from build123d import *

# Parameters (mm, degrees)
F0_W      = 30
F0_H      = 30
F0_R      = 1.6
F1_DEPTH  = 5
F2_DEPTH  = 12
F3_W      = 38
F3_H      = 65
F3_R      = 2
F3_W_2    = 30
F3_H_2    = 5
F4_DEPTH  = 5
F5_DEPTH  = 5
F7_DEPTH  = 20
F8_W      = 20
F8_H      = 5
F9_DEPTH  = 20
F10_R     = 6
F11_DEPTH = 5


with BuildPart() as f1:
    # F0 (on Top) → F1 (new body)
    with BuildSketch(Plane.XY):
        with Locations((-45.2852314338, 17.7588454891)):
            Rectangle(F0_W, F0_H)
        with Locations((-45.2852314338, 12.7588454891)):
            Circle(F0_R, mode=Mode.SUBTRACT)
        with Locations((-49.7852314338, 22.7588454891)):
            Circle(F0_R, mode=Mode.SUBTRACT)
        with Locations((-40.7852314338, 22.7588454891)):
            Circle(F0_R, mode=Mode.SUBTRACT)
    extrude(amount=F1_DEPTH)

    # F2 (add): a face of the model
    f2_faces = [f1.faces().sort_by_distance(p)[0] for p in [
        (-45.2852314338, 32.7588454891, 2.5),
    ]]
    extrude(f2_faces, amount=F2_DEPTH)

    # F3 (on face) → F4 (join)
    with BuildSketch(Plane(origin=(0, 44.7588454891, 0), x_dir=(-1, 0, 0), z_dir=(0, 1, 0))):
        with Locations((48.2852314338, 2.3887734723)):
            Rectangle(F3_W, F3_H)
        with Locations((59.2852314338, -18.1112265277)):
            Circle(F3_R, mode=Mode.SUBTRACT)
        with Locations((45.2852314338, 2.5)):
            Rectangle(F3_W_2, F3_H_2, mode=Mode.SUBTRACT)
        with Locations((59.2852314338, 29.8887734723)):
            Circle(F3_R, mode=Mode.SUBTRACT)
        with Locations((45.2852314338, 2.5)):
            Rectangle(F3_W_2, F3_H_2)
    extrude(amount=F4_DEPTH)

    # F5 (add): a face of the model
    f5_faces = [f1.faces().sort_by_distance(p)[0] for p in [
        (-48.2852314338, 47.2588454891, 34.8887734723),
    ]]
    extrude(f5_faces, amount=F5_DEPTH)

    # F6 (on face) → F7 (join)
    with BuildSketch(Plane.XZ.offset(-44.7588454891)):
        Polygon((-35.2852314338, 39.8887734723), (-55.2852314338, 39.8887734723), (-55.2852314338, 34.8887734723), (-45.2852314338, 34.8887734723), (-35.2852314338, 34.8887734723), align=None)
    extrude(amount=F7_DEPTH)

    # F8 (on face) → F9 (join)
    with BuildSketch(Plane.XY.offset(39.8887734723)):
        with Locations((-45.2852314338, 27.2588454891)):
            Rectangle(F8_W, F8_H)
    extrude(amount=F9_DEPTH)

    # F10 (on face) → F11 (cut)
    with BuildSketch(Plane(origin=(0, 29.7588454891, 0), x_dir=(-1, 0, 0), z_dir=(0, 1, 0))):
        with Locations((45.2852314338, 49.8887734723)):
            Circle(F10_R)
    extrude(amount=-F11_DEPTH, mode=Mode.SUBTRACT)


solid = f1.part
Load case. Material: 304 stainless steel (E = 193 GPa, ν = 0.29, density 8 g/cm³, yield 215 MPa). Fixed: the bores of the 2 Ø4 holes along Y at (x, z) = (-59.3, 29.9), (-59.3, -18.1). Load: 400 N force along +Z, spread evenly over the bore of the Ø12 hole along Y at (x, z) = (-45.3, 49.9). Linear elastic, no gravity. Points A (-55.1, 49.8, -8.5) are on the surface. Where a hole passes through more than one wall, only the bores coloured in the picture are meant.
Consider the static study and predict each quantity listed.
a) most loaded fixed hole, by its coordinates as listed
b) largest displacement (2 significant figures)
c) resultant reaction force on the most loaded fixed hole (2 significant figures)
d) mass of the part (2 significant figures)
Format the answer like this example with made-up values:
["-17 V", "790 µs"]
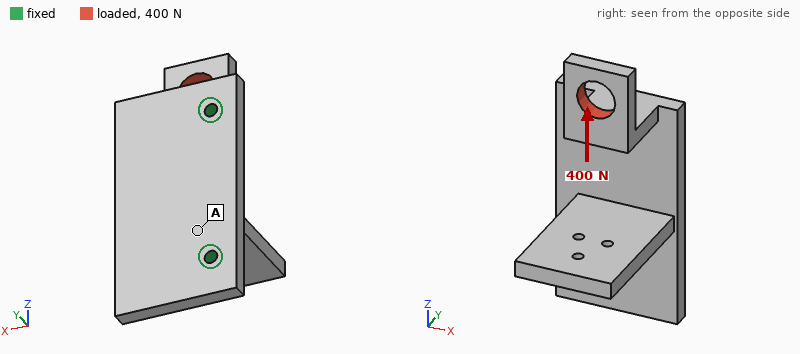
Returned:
["(-59.3, 29.9)", "0.11 mm", "290 N", "180 g"]
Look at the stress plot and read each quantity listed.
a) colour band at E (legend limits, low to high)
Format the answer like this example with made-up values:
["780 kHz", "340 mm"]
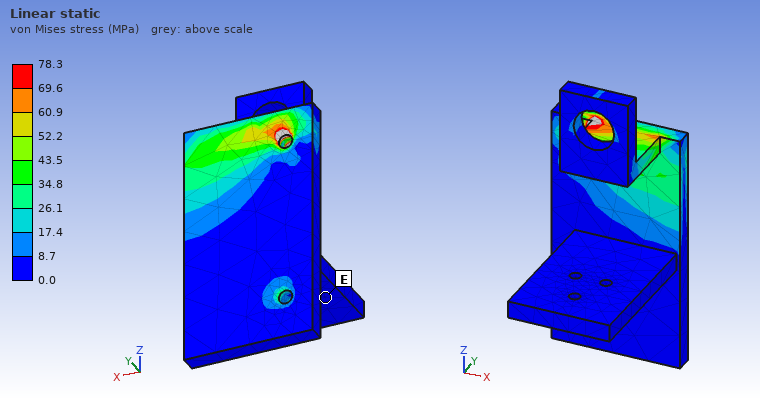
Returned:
["0.0 to 8.7 MPa"]
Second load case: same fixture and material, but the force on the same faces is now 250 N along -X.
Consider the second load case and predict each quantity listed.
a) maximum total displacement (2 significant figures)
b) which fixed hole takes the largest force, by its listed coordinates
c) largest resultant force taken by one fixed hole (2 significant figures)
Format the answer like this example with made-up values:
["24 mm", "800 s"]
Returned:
["45 µm", "(-59.3, 29.9)", "360 N"]
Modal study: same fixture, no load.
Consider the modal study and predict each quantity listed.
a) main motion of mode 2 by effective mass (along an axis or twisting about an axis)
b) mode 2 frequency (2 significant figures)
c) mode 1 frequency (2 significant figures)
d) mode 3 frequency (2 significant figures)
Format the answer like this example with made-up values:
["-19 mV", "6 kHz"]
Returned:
["along Z", "1900 Hz", "1800 Hz", "2300 Hz"]
